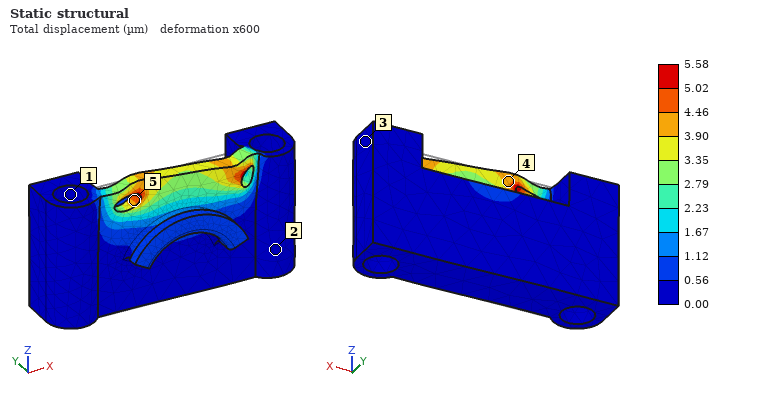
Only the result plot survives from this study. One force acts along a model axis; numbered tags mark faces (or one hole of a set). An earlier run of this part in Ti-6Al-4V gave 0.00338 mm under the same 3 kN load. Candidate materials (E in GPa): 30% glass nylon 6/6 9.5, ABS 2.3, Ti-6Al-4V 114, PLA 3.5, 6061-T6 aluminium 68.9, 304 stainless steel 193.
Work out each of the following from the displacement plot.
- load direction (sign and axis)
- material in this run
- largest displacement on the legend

+X
6061-T6 aluminium
5.58 µm
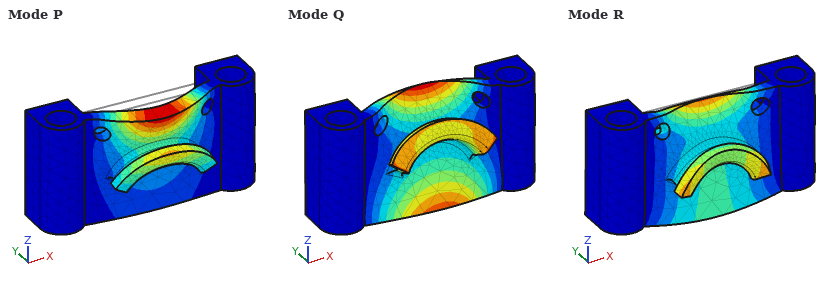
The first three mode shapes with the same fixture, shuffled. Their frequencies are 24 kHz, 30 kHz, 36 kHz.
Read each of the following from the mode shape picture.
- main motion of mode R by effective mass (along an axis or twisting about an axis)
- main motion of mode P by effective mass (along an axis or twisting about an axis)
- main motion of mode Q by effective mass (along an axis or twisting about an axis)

along Z
along Y
along Y
